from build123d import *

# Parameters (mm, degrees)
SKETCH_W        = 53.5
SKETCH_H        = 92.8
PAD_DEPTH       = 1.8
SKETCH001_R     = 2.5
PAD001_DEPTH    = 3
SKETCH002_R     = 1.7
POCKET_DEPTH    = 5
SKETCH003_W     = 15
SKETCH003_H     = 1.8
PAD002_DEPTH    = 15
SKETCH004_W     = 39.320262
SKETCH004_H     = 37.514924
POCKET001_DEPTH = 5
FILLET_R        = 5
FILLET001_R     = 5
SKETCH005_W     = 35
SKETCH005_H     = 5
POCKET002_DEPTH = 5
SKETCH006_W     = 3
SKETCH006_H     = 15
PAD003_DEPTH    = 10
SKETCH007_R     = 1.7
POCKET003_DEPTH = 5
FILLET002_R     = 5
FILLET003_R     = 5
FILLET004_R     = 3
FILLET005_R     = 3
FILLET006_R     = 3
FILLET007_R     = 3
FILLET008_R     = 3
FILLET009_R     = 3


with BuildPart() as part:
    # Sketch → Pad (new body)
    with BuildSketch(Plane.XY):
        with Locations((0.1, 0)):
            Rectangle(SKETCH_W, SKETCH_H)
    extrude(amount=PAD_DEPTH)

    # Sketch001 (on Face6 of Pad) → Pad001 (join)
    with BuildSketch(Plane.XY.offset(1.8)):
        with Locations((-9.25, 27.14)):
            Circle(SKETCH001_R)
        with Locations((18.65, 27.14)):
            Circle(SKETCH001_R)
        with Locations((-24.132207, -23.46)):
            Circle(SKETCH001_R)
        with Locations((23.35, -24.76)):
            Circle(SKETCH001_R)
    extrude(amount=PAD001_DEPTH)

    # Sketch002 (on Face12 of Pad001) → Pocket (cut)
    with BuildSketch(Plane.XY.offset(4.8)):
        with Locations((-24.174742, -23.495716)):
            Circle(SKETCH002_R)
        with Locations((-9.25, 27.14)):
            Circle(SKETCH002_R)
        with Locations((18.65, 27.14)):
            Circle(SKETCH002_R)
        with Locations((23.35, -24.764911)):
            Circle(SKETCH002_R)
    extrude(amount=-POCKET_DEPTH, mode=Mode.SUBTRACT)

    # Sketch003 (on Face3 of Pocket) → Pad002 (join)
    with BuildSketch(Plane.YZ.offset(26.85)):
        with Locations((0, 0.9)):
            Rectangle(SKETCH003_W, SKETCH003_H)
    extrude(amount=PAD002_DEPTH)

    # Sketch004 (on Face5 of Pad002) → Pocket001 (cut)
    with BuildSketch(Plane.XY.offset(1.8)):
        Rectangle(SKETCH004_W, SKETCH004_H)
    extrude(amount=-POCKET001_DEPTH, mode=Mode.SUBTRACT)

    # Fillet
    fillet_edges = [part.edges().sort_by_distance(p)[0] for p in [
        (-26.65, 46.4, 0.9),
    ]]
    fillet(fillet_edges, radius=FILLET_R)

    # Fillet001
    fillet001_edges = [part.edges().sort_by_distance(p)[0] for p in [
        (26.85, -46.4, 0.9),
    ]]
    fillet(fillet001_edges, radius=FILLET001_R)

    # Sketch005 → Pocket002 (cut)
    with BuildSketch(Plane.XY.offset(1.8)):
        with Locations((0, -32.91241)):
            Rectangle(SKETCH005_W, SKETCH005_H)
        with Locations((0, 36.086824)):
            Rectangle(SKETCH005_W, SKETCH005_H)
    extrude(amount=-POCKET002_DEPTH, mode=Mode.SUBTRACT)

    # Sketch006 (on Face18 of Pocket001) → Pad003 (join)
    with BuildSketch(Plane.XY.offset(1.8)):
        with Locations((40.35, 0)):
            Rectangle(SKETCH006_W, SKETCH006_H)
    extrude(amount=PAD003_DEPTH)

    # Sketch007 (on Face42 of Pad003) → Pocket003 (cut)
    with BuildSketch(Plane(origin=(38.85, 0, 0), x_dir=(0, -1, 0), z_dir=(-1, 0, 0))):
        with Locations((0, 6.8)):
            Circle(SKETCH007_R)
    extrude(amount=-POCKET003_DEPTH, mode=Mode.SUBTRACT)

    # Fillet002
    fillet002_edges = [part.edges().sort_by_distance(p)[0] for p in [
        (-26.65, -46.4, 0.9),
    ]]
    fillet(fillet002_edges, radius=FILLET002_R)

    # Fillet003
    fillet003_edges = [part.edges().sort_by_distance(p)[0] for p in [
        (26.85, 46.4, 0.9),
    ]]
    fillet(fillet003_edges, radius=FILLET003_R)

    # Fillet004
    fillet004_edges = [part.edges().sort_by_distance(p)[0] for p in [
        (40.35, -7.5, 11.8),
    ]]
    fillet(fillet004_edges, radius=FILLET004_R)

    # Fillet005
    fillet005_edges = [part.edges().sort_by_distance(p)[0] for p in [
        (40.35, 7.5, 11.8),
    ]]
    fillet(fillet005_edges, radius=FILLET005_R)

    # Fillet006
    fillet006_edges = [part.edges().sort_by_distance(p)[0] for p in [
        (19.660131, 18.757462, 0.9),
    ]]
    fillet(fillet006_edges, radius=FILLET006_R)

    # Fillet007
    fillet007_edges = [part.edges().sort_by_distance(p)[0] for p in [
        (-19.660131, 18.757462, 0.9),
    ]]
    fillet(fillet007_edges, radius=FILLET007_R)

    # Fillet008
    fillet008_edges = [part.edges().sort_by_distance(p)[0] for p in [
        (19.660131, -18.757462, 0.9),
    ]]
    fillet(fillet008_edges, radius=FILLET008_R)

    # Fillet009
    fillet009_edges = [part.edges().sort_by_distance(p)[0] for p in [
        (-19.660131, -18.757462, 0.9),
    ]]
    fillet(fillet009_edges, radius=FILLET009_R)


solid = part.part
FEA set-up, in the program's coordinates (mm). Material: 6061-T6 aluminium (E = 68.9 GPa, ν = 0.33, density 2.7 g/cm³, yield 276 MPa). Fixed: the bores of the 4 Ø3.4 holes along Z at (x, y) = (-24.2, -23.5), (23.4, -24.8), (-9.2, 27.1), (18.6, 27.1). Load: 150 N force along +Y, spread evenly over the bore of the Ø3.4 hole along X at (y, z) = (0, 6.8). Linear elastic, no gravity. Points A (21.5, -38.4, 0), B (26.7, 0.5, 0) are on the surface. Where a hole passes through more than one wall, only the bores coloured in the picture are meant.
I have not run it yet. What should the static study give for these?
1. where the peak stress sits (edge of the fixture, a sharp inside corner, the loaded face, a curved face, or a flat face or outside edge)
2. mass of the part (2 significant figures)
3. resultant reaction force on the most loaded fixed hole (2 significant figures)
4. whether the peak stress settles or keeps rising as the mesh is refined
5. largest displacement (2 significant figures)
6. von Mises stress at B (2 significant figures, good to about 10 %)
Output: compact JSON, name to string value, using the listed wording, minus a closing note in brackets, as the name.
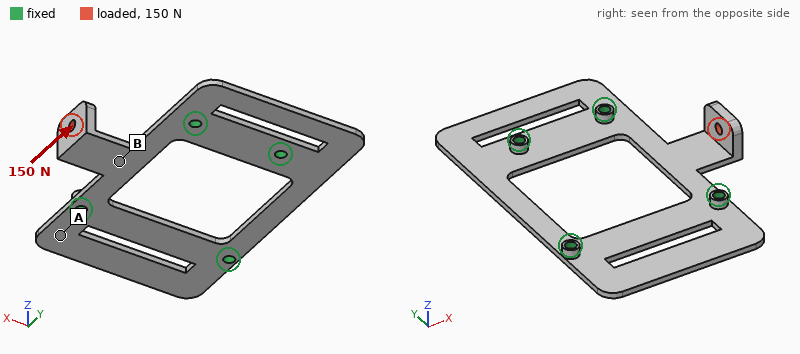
{"where the peak stress sits": "a sharp inside corner", "mass of the part": "18 g", "resultant reaction force on the most loaded fixed hole": "97 N", "whether the peak stress settles or keeps rising as the mesh is refined": "keeps rising", "largest displacement": "0.25 mm", "von Mises stress at B": "61 MPa"}
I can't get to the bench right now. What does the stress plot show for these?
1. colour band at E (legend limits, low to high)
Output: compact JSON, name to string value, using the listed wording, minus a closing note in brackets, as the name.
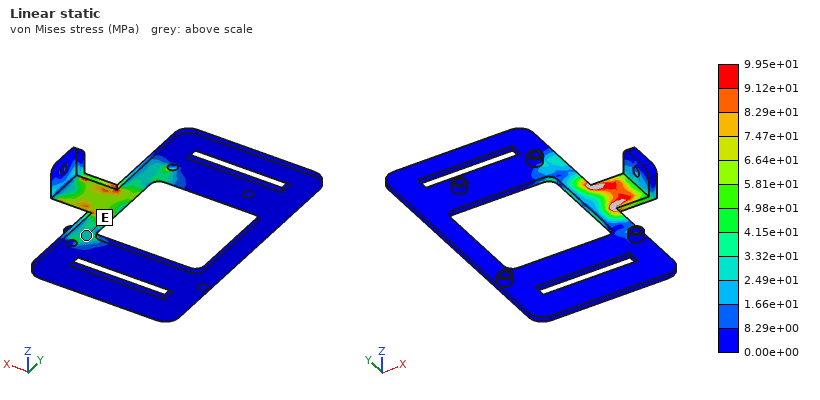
{"colour band at E": "2.49e+01 to 3.32e+01 MPa"}
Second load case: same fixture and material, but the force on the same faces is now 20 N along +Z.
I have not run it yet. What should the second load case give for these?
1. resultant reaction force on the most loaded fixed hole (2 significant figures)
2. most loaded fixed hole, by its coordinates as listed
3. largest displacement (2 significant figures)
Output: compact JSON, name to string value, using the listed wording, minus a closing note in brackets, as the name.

{"resultant reaction force on the most loaded fixed hole": "12 N", "most loaded fixed hole, by its coordinates as listed": "(23.4, -24.8)", "largest displacement": "0.31 mm"}
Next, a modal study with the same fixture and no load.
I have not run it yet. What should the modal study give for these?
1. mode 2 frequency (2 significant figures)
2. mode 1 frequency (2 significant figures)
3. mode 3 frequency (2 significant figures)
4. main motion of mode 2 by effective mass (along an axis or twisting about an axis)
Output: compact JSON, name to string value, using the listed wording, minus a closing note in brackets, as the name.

{"mode 2 frequency": "1900 Hz", "mode 1 frequency": "1100 Hz", "mode 3 frequency": "2300 Hz", "main motion of mode 2 by effective mass": "along Z"}
